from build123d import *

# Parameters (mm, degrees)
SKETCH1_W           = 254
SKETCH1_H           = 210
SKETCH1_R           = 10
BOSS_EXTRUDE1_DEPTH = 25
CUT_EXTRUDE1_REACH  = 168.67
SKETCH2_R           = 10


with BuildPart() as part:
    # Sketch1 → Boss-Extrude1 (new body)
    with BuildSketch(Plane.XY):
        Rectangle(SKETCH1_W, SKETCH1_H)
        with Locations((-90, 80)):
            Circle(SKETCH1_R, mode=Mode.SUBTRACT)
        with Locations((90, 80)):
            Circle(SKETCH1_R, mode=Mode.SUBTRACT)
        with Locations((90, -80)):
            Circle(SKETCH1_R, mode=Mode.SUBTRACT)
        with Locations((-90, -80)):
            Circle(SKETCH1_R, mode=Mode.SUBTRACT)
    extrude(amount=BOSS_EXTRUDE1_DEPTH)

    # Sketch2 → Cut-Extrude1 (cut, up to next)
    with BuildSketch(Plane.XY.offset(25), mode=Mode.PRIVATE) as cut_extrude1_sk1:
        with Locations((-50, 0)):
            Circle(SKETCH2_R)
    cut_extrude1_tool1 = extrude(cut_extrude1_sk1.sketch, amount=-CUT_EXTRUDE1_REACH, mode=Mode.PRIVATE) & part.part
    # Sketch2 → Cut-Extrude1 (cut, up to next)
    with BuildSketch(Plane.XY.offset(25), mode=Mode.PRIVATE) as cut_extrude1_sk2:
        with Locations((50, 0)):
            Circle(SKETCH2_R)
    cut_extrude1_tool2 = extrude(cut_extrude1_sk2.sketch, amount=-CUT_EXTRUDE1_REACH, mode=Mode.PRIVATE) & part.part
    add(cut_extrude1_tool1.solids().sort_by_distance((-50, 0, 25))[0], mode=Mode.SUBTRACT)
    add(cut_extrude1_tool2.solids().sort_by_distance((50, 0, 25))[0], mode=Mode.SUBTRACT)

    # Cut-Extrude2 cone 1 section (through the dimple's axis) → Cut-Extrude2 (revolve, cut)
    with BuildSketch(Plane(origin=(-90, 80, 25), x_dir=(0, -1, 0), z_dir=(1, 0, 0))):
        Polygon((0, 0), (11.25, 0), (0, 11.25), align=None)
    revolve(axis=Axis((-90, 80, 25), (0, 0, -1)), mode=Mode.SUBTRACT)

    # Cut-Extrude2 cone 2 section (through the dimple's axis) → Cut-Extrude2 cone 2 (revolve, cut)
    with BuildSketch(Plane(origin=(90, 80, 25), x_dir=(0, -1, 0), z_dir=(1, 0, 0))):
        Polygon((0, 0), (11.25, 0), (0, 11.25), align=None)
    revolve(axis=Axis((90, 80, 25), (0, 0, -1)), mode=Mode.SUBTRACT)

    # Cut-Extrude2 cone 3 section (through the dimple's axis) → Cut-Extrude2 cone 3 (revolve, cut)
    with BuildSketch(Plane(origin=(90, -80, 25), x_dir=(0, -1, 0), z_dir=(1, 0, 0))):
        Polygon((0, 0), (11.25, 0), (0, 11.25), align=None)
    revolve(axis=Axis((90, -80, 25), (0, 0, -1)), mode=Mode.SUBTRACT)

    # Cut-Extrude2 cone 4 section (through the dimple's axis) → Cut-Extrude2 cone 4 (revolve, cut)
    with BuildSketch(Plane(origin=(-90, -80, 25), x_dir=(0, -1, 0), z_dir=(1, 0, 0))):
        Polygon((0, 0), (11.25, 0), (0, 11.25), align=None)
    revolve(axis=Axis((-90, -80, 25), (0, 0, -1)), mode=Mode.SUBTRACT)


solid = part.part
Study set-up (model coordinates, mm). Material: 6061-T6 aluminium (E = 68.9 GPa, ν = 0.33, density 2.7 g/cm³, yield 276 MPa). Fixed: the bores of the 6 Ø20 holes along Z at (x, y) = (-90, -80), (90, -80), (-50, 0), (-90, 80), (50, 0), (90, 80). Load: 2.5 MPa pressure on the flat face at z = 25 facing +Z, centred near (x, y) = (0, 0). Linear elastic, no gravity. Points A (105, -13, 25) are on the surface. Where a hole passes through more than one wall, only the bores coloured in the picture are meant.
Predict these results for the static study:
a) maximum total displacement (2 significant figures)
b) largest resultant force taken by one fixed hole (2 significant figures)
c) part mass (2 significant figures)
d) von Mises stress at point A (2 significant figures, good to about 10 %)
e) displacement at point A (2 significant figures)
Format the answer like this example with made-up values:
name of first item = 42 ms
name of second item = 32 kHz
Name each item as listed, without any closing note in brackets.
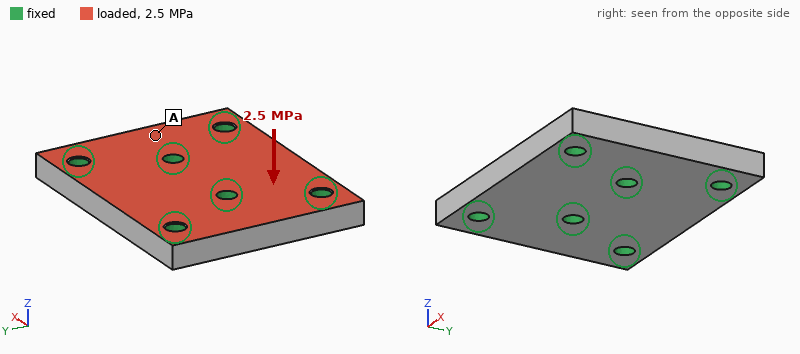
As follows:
maximum total displacement = 71 µm
largest resultant force taken by one fixed hole = 26 kN
part mass = 3.5 kg
von Mises stress at point A = 7.9 MPa
displacement at point A = 25 µm
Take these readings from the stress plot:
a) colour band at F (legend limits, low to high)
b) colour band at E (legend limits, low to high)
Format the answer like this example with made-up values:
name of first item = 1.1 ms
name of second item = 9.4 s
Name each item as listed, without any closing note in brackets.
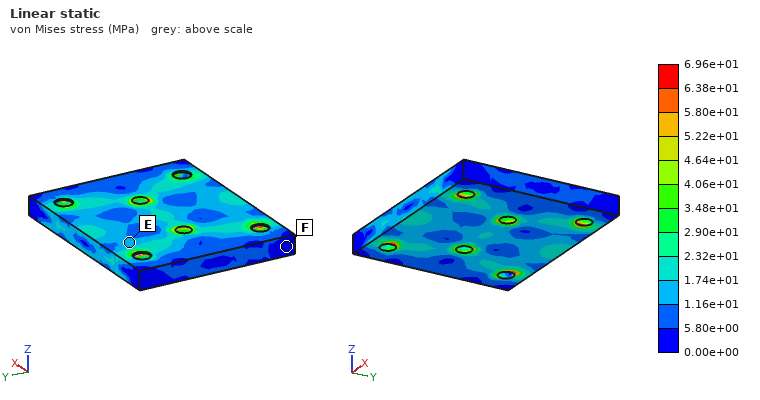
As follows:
colour band at F = 0.00e+00 to 5.80e+00 MPa
colour band at E = 1.16e+01 to 1.74e+01 MPa
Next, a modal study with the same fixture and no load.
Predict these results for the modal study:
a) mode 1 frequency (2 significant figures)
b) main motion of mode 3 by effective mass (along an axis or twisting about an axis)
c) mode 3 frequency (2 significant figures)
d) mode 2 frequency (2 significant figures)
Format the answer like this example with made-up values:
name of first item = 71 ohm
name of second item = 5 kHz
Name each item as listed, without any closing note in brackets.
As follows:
mode 1 frequency = 4600 Hz
main motion of mode 3 by effective mass = twisting about Y
mode 3 frequency = 5900 Hz
mode 2 frequency = 4600 Hz
